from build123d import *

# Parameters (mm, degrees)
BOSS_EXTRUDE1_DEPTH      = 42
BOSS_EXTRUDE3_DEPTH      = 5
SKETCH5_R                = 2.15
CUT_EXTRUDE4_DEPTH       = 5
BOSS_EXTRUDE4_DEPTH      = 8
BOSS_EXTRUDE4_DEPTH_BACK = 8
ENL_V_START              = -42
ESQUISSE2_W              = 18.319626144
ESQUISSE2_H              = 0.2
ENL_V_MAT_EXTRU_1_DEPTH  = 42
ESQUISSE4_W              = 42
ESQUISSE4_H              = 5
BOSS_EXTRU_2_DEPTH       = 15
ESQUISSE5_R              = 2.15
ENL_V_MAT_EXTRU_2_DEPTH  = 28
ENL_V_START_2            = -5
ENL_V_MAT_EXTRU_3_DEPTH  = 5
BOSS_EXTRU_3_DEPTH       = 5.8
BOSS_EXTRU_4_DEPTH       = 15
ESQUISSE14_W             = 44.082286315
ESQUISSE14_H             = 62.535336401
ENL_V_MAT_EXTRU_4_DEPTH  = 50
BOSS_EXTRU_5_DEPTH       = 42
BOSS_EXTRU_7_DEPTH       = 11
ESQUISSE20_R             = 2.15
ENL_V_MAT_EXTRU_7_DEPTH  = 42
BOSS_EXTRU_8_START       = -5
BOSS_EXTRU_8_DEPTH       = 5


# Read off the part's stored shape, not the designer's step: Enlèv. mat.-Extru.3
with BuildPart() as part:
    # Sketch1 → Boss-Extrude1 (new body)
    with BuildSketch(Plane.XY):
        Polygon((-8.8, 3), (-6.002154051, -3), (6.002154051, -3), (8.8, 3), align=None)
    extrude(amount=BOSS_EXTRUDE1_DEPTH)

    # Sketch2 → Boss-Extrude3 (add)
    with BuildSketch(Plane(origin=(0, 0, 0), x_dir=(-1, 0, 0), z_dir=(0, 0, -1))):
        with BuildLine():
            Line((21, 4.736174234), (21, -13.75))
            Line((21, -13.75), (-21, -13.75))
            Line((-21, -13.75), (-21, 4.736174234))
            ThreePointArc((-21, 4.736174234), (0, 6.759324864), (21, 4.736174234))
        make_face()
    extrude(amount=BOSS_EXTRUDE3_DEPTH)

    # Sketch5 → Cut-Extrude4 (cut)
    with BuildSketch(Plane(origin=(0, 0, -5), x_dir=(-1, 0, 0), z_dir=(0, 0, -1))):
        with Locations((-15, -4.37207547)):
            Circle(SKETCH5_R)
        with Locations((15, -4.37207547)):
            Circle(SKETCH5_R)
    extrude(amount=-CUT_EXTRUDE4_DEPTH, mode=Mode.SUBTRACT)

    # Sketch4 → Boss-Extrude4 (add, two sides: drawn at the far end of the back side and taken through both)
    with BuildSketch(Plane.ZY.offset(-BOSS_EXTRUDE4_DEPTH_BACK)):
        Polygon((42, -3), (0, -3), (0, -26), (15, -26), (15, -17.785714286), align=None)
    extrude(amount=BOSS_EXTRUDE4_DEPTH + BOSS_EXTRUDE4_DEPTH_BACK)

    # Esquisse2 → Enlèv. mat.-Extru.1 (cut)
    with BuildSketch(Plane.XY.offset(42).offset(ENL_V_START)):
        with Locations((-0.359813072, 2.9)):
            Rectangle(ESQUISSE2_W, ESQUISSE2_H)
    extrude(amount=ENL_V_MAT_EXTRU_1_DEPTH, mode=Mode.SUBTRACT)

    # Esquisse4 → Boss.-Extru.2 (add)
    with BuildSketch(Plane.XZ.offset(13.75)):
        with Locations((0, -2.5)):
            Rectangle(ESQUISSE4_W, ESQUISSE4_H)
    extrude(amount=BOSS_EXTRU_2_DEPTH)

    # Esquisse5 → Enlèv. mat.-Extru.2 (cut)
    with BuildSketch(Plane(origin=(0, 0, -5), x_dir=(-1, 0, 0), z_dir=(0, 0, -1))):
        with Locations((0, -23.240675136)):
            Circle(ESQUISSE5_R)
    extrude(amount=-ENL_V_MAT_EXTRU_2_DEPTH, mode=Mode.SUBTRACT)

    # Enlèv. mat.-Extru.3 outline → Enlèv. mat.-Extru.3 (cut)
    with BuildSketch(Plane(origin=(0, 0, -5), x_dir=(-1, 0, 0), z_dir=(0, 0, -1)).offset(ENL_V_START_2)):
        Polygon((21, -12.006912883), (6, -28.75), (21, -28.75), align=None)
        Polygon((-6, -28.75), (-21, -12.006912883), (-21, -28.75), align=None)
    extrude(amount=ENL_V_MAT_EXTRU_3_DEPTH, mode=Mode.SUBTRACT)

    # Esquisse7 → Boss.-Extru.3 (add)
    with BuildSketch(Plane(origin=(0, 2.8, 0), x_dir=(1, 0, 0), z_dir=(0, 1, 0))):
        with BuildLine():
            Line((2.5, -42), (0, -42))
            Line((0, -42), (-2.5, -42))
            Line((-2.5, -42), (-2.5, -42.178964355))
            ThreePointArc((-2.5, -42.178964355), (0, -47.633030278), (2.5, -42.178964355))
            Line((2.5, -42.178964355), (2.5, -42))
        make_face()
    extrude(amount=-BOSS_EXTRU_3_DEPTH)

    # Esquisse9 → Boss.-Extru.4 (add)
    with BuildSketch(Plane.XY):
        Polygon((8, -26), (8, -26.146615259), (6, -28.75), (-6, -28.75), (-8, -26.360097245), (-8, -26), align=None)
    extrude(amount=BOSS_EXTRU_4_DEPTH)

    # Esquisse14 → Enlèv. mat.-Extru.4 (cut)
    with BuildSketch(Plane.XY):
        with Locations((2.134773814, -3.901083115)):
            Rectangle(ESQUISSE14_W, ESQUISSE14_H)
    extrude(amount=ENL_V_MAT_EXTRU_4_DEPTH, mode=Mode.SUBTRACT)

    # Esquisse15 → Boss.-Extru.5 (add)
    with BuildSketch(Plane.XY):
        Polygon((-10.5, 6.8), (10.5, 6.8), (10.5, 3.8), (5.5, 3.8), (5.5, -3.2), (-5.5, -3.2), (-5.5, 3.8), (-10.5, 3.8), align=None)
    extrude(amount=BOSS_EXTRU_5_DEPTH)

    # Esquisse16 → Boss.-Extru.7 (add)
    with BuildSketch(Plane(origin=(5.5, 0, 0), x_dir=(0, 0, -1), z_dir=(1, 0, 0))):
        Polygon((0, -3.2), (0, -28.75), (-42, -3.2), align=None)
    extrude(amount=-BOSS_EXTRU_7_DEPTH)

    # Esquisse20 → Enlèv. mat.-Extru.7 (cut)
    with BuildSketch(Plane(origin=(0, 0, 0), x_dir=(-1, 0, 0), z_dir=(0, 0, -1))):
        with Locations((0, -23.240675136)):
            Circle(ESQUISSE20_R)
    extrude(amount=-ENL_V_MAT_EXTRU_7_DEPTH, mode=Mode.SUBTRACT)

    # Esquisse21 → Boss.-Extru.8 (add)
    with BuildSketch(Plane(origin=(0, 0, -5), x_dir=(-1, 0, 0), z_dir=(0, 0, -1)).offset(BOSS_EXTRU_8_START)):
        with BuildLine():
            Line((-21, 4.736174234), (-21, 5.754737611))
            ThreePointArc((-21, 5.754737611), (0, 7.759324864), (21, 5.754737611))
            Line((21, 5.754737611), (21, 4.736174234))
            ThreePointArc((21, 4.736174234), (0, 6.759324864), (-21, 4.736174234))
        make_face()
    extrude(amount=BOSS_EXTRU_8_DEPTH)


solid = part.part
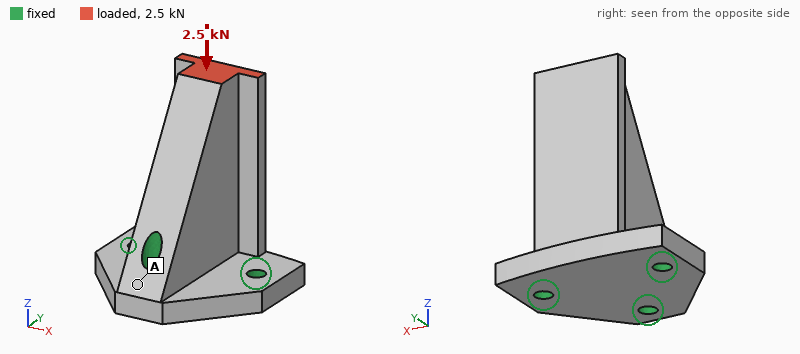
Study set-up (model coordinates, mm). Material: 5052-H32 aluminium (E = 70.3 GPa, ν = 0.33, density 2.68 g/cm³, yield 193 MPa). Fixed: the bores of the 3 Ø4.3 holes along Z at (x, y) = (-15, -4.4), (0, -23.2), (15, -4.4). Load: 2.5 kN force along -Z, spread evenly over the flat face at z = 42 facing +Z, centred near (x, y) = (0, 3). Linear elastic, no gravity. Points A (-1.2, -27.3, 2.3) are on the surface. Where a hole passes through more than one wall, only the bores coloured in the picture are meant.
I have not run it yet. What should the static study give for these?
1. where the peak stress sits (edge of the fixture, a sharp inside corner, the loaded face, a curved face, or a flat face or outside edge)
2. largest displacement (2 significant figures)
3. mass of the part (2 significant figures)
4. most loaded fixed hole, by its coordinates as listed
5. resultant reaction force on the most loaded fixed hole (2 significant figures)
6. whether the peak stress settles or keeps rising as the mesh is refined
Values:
edge of the fixture
44 µm
47 g
(0, -23.2)
1.3 kN
keeps rising
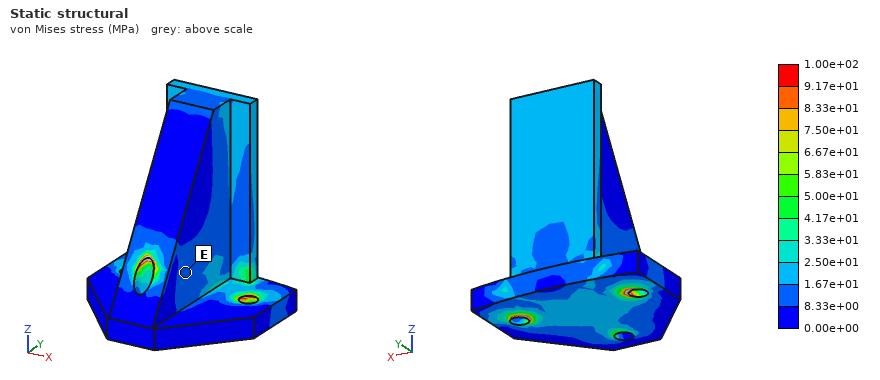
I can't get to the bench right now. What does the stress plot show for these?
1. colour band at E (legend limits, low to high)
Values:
8.33e+00 to 1.67e+01 MPa
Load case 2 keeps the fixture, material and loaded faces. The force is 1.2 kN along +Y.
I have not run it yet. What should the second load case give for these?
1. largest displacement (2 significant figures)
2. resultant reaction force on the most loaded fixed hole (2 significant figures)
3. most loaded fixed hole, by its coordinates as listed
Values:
58 µm
2.3 kN
(0, -23.2)
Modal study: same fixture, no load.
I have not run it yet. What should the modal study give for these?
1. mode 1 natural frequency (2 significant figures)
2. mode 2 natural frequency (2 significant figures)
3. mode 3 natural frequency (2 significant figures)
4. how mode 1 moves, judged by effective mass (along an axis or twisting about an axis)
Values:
5600 Hz
9100 Hz
19 kHz
along X
